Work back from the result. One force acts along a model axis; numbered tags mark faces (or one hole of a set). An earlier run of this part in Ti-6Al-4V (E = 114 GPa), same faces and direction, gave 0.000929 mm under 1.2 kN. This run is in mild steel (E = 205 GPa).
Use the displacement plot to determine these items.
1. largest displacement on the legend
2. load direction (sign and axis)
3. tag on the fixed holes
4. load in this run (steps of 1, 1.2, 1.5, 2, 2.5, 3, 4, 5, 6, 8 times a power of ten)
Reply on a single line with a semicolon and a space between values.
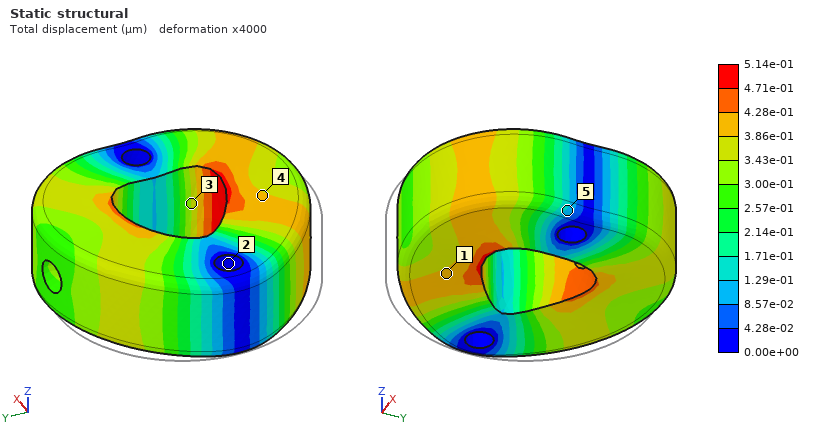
5.14e-01 µm; +X; 2; 1.2 kN
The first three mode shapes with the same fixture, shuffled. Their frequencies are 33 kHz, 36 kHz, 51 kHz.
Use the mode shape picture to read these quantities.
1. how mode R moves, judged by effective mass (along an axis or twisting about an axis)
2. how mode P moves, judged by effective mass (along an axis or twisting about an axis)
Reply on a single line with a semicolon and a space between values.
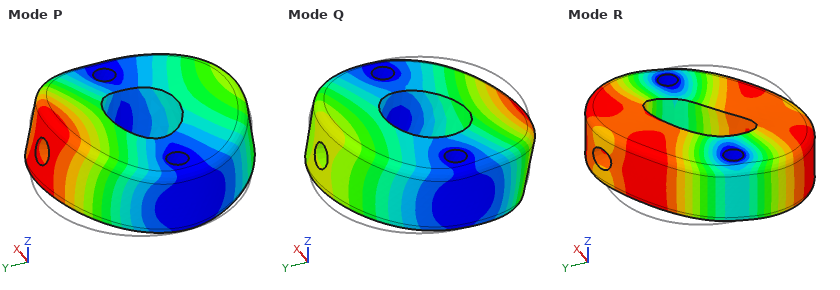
twisting about Z; along Z
